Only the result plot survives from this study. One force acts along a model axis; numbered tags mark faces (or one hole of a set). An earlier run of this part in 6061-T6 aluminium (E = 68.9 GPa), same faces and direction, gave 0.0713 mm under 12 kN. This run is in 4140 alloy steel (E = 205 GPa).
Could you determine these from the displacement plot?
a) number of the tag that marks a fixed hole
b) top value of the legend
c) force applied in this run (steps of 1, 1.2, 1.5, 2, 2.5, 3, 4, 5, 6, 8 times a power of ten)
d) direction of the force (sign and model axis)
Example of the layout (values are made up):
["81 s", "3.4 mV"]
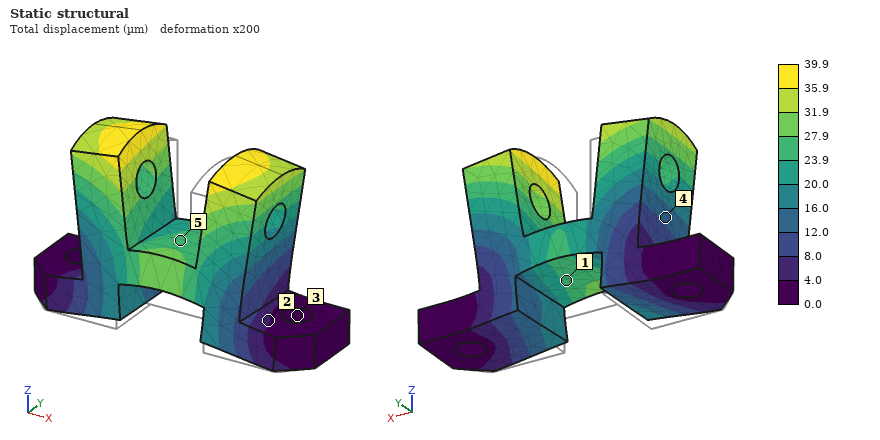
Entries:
["3", "39.9 µm", "20 kN", "+Z"]
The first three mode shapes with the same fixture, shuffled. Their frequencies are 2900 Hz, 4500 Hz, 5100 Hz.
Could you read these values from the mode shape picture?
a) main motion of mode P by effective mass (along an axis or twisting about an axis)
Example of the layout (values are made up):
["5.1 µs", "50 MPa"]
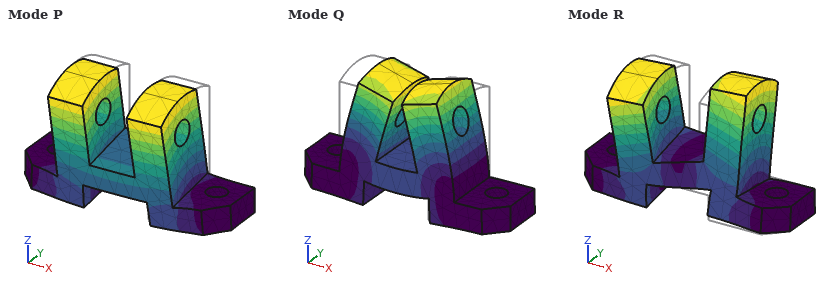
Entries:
["along Y"]
